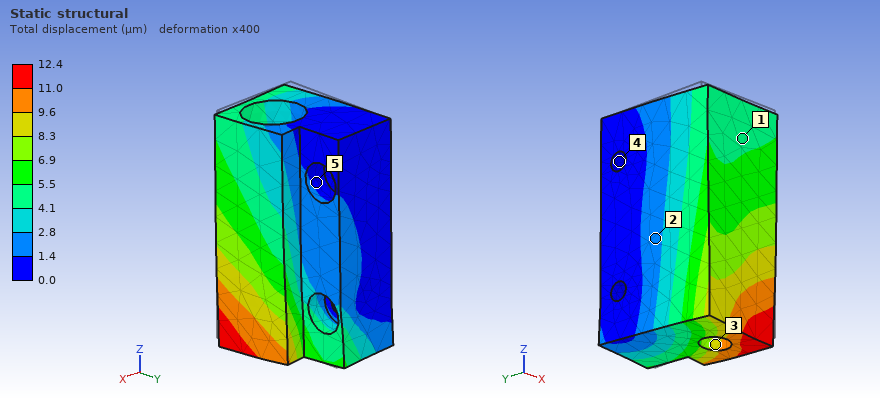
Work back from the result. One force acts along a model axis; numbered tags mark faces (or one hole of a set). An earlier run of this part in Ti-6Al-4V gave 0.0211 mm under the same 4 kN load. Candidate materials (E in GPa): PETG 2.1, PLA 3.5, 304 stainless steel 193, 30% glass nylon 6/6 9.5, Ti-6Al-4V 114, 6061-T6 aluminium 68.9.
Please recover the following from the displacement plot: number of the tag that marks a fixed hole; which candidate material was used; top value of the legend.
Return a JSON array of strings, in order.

["4", "304 stainless steel", "12.4 µm"]
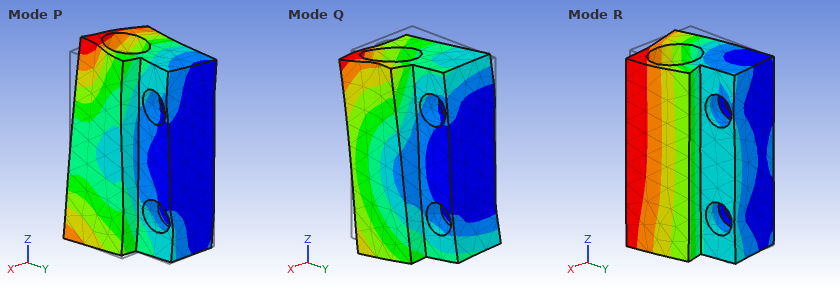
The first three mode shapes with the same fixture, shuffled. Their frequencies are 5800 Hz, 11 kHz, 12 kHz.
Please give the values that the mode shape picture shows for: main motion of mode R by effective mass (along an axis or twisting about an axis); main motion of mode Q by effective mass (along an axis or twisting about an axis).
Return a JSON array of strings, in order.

["along X", "along Z"]
